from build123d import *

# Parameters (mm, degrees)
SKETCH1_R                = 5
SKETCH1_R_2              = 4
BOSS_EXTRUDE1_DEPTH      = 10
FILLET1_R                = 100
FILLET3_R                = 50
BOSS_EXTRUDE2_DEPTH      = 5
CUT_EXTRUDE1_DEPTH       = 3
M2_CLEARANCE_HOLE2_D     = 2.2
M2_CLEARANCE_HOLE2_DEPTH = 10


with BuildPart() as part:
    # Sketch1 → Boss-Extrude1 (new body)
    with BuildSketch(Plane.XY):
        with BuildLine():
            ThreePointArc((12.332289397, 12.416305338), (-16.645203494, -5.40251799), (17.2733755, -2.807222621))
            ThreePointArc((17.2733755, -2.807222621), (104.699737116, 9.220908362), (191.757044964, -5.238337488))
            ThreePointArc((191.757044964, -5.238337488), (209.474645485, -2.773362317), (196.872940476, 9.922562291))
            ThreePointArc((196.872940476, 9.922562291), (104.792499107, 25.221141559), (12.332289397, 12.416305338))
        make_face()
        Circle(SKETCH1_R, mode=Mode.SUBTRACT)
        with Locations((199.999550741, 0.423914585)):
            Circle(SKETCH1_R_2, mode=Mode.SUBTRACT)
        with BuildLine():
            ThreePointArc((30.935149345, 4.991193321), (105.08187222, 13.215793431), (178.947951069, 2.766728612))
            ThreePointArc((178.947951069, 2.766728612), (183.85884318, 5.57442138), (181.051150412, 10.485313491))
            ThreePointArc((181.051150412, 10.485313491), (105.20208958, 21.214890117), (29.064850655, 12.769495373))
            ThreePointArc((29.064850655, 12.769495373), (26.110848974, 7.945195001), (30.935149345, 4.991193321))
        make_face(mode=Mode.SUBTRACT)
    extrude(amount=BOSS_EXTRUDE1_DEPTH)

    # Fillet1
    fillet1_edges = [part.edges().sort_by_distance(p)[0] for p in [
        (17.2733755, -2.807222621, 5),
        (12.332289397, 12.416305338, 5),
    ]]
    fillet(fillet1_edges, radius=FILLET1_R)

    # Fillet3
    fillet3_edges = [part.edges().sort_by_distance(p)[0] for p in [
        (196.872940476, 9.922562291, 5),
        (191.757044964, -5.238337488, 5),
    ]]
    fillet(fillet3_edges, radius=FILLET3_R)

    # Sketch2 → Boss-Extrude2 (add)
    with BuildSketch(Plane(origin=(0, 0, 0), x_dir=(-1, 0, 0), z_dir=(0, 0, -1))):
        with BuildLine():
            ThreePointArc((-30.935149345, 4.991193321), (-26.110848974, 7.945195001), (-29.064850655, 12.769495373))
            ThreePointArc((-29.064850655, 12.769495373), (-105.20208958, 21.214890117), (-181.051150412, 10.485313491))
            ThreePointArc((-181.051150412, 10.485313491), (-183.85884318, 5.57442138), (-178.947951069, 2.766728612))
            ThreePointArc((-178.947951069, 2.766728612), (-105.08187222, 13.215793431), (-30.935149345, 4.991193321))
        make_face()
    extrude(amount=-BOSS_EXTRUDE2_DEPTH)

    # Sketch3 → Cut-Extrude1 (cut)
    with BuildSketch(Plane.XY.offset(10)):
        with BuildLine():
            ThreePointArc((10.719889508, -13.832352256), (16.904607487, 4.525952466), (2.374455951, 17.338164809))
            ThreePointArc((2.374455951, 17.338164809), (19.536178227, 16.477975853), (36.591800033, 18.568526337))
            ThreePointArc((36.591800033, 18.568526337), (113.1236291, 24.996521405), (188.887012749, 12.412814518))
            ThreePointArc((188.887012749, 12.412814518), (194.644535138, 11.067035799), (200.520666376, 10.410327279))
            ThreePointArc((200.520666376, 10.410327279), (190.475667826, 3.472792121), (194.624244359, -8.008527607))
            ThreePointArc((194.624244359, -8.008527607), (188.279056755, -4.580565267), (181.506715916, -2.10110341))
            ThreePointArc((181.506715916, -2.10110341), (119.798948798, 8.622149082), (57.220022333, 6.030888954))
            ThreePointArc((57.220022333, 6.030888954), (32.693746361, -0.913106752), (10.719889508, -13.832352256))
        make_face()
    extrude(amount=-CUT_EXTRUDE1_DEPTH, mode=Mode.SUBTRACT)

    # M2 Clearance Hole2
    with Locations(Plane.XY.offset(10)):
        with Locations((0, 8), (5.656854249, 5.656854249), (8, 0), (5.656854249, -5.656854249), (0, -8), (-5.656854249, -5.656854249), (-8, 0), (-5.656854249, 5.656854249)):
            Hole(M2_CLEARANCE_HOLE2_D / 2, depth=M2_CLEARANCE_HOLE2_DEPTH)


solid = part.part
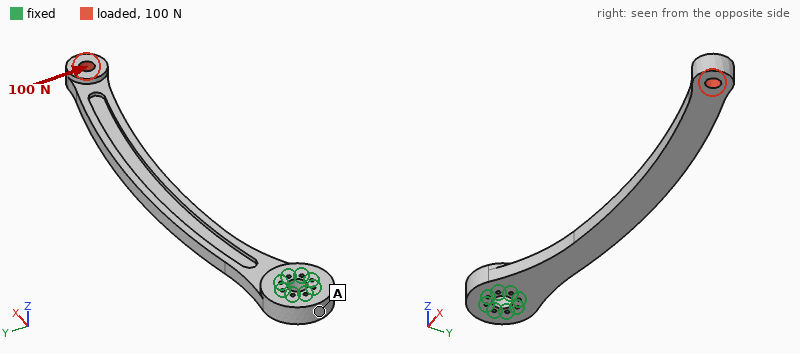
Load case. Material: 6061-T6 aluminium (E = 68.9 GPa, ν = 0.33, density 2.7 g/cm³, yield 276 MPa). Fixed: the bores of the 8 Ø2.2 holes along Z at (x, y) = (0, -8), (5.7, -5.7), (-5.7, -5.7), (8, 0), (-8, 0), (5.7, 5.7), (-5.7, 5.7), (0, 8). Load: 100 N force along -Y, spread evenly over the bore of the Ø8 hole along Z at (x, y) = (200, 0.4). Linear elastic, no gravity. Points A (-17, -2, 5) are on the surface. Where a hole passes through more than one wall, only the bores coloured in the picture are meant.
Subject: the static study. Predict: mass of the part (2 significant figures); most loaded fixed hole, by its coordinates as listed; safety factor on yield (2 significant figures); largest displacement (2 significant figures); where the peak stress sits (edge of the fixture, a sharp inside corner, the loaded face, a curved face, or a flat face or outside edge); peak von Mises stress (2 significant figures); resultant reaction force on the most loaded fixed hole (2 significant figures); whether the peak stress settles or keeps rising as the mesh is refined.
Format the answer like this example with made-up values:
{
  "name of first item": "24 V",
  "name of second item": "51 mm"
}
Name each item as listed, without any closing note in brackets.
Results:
{
  "mass of the part": "80 g",
  "most loaded fixed hole, by its coordinates as listed": "(5.7, -5.7)",
  "safety factor on yield": "5.1",
  "largest displacement": "1.3 mm",
  "where the peak stress sits": "a curved face",
  "peak von Mises stress": "54 MPa",
  "resultant reaction force on the most loaded fixed hole": "610 N",
  "whether the peak stress settles or keeps rising as the mesh is refined": "settles"
}
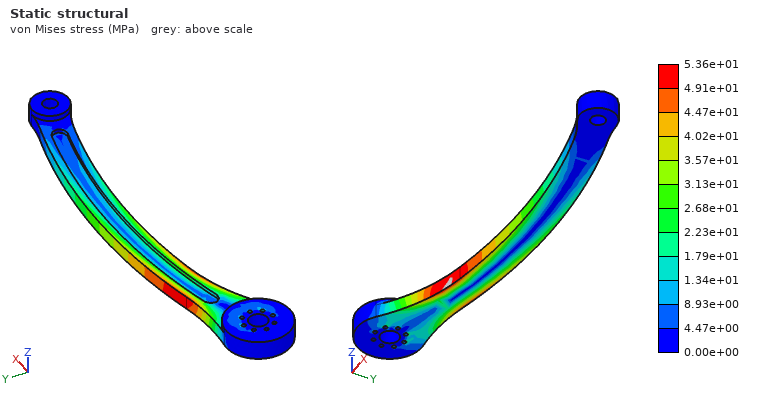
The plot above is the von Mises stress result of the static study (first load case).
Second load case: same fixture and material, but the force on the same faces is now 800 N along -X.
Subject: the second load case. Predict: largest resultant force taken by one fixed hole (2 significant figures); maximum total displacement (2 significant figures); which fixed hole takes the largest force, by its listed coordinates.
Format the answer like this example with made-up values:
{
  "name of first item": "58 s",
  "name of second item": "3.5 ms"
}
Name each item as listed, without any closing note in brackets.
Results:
{
  "largest resultant force taken by one fixed hole": "260 N",
  "maximum total displacement": "1.6 mm",
  "which fixed hole takes the largest force, by its listed coordinates": "(8, 0)"
}
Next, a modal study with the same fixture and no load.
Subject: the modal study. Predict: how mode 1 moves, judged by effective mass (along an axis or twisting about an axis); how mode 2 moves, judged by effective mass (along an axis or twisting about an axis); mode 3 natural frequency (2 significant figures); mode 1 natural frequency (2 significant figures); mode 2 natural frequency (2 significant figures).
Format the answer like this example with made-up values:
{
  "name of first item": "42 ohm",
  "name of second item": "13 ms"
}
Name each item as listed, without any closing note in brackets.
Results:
{
  "how mode 1 moves, judged by effective mass": "along Z",
  "how mode 2 moves, judged by effective mass": "along Y",
  "mode 3 natural frequency": "780 Hz",
  "mode 1 natural frequency": "130 Hz",
  "mode 2 natural frequency": "360 Hz"
}
